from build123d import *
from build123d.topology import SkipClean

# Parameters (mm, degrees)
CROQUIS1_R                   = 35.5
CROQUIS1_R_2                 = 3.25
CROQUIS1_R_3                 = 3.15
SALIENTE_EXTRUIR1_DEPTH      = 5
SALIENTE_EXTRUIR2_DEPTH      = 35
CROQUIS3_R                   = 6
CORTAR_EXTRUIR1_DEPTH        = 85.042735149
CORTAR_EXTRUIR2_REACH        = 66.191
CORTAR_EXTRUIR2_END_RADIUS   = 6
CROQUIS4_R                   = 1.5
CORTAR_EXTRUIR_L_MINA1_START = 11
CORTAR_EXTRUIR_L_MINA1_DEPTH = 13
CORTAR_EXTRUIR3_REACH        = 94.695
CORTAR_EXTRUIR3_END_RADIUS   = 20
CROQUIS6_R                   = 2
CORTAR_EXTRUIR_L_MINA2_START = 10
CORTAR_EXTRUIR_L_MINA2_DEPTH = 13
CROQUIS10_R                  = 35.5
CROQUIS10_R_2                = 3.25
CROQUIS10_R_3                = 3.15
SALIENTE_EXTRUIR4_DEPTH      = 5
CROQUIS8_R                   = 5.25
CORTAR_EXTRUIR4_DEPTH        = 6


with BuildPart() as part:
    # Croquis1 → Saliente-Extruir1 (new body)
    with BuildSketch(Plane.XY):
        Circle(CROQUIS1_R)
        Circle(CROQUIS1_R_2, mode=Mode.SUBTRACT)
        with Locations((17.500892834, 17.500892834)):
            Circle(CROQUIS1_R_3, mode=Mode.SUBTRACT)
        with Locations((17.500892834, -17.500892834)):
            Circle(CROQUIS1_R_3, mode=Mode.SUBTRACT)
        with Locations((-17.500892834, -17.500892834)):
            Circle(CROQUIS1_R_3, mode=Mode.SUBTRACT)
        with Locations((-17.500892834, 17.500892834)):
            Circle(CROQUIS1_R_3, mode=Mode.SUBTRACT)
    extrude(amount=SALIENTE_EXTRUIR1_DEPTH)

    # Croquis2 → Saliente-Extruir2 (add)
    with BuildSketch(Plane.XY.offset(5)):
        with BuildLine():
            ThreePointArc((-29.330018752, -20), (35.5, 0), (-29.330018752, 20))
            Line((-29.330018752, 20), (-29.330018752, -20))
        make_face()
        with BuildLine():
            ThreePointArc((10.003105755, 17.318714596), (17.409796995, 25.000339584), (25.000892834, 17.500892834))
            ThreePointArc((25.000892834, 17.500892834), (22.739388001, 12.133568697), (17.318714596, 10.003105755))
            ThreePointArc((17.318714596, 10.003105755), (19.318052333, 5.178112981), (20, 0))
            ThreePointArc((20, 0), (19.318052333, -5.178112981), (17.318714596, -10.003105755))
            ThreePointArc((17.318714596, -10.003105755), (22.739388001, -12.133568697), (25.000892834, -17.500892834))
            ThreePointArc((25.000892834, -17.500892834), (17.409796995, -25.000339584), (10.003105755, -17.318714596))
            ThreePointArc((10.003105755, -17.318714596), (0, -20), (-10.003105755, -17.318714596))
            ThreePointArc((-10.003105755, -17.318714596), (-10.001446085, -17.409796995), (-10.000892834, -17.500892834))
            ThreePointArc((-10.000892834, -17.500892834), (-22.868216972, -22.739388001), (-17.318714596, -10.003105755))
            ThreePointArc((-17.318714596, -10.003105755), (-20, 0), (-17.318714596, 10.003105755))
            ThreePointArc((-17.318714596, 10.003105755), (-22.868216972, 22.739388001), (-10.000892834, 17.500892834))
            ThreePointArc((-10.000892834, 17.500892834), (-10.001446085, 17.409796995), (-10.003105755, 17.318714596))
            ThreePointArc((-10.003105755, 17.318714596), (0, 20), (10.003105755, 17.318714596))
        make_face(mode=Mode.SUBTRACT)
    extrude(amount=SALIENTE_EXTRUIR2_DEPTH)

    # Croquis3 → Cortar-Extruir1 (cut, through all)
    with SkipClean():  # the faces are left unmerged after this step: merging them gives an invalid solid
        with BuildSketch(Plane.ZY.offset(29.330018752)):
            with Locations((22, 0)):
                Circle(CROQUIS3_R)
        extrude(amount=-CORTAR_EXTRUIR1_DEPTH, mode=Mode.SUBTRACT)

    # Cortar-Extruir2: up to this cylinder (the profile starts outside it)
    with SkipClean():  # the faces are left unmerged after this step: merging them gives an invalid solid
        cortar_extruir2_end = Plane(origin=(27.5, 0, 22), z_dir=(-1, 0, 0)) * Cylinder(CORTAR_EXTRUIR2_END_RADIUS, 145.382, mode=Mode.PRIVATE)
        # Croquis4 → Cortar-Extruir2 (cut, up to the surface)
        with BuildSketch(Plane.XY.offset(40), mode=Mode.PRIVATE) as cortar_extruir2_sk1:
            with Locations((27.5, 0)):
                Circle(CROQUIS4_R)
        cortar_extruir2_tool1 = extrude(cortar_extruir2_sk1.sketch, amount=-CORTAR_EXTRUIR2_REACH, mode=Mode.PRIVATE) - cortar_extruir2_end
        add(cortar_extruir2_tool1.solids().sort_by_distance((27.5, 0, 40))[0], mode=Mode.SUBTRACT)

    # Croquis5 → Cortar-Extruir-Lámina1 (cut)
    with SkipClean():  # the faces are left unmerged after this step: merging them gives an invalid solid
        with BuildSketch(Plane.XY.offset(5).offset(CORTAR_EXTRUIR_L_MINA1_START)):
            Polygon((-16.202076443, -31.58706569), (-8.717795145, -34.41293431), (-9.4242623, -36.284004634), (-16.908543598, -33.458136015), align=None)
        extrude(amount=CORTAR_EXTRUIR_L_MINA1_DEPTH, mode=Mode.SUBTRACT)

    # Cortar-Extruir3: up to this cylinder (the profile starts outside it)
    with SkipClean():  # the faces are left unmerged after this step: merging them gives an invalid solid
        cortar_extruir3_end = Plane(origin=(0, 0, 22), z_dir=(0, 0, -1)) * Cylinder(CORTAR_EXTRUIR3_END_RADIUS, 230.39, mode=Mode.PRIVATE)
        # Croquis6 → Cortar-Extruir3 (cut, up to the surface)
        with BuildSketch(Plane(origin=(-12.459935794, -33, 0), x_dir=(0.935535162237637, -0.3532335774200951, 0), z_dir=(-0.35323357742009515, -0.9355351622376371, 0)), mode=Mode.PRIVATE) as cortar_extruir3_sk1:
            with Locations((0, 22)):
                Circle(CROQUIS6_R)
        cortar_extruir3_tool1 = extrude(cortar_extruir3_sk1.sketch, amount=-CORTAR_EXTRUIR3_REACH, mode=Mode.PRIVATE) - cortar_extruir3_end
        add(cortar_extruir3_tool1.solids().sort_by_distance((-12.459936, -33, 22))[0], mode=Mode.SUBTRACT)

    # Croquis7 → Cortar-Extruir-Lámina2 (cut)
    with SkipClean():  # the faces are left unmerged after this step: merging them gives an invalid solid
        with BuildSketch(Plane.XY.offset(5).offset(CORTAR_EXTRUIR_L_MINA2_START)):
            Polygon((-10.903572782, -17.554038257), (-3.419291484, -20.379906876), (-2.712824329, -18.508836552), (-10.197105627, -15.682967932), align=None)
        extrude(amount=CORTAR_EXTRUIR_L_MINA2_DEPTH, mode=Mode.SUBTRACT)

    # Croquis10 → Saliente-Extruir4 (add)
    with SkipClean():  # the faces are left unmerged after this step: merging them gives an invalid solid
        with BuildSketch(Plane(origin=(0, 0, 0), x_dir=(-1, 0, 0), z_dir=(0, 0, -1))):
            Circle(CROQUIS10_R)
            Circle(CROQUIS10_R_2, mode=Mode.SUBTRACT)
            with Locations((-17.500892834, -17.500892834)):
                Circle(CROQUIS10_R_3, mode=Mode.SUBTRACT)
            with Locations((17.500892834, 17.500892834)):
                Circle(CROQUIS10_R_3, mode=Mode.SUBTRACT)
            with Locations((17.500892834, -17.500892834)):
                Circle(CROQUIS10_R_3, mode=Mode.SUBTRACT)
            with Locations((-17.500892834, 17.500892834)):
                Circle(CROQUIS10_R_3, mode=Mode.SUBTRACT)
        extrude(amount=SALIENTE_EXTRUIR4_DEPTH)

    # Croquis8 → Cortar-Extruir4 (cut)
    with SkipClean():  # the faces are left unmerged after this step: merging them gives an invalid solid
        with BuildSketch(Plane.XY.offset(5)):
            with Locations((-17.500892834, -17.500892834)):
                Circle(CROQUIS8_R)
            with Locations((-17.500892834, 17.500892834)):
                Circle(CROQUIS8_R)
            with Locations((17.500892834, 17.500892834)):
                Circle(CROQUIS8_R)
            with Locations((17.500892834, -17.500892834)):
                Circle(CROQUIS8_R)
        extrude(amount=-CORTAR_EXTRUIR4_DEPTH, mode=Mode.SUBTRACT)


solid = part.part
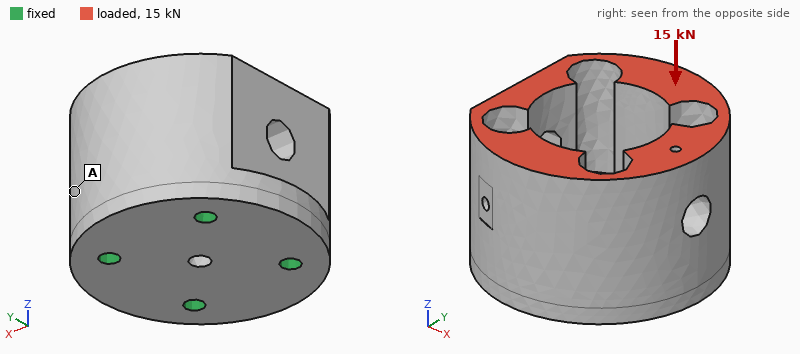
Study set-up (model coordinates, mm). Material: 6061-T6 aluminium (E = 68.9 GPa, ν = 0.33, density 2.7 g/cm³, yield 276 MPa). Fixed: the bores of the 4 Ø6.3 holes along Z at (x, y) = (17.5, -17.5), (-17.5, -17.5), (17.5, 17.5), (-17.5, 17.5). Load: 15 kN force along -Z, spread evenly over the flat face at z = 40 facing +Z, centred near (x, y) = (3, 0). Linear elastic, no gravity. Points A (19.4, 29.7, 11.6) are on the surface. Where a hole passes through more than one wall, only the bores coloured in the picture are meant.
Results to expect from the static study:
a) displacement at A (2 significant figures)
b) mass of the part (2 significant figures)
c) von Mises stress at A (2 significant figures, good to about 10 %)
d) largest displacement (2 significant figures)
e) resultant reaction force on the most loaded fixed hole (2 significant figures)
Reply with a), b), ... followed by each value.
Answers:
a) 13 µm
b) 270 g
c) 15 MPa
d) 19 µm
e) 4.3 kN
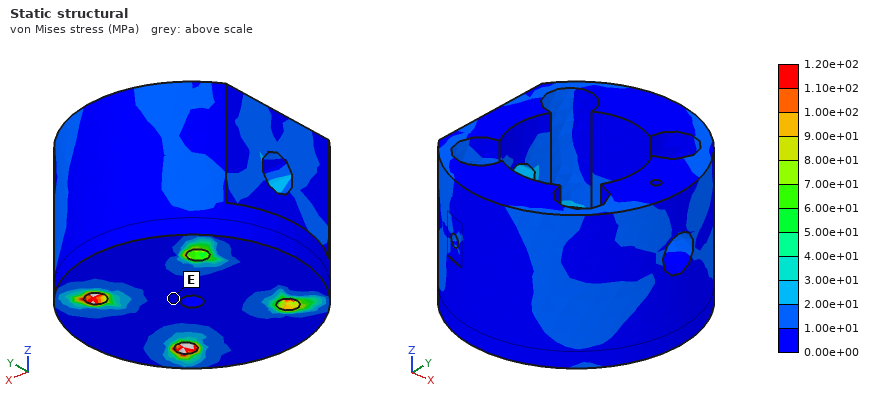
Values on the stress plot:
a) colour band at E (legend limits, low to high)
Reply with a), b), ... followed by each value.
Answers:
a) 0.00e+00 to 1.00e+01 MPa
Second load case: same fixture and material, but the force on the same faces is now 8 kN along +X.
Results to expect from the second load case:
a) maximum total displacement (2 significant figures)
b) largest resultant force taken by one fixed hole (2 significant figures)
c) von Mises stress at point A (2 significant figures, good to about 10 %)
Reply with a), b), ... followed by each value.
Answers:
a) 0.11 mm
b) 5.1 kN
c) 22 MPa
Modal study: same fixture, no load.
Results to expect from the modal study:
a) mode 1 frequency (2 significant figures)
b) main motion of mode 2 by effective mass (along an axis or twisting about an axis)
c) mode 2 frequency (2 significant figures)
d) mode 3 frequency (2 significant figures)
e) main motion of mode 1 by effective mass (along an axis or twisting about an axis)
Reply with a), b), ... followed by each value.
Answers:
a) 5500 Hz
b) along X
c) 6000 Hz
d) 6800 Hz
e) along Y
